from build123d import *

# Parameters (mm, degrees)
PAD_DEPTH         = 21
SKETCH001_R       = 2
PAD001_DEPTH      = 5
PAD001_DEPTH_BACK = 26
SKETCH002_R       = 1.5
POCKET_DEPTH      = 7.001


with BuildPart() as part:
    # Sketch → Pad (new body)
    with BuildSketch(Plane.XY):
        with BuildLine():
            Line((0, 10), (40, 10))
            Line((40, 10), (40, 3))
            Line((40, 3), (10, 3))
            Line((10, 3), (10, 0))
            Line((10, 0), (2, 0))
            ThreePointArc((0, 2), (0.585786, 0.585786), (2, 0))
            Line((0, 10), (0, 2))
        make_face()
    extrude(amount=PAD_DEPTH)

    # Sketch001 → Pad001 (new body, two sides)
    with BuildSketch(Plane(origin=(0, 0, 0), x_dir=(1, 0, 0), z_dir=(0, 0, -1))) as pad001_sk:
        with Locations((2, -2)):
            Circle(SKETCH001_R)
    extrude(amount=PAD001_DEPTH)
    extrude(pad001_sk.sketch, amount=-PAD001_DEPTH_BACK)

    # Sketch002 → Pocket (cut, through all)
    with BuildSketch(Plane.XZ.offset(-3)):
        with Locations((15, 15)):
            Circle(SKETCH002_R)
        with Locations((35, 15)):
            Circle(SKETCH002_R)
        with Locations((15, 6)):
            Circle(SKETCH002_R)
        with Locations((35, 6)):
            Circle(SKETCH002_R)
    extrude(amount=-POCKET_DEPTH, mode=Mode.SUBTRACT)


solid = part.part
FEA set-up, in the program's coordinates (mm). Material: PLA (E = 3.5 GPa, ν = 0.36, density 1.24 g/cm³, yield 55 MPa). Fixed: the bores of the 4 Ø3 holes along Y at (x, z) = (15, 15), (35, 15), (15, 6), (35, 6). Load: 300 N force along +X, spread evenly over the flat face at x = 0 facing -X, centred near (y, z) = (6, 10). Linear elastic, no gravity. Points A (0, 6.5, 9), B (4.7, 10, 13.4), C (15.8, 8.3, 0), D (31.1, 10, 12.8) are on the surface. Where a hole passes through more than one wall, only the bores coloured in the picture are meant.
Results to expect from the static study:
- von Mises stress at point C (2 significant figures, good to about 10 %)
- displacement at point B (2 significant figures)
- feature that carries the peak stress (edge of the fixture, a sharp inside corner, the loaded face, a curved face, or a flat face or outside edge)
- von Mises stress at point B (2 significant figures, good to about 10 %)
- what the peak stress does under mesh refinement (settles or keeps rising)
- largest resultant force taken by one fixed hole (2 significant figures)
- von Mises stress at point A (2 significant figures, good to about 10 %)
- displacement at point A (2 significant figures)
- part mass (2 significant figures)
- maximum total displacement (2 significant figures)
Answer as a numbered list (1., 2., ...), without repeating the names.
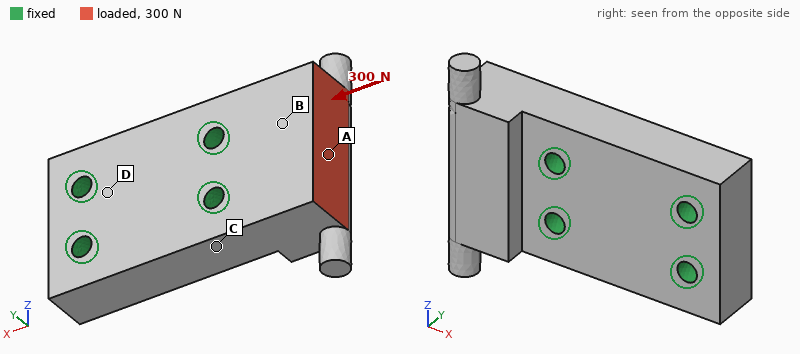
1. 1.0 MPa
2. 5.2 µm
3. edge of the fixture
4. 2.1 MPa
5. keeps rising
6. 140 N
7. 1.7 MPa
8. 9.2 µm
9. 8.0 g
10. 11 µm
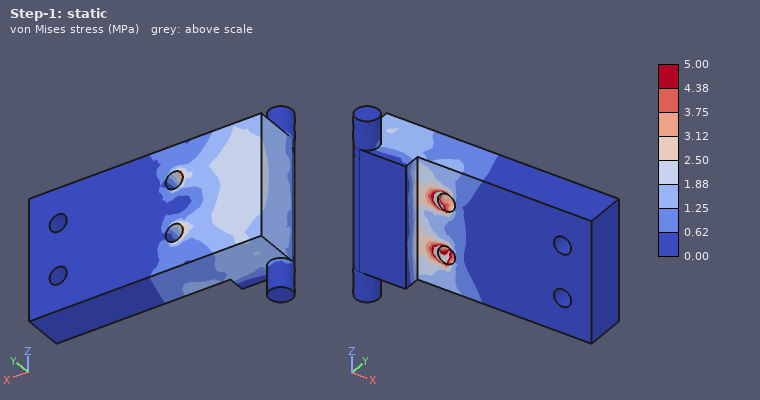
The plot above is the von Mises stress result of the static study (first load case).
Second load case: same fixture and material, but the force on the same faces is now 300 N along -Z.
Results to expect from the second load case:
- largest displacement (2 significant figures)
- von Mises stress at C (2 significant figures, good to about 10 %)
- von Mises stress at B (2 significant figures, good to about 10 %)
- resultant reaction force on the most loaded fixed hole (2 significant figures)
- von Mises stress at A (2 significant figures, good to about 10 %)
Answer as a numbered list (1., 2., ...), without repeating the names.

1. 69 µm
2. 5.9 MPa
3. 5.6 MPa
4. 340 N
5. 3.3 MPa
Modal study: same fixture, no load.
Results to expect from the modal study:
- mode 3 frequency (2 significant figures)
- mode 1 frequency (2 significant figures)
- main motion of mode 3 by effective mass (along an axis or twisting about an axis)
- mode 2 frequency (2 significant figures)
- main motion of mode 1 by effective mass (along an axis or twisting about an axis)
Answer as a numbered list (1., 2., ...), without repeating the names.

1. 9500 Hz
2. 5900 Hz
3. along Z
4. 8700 Hz
5. along Y
